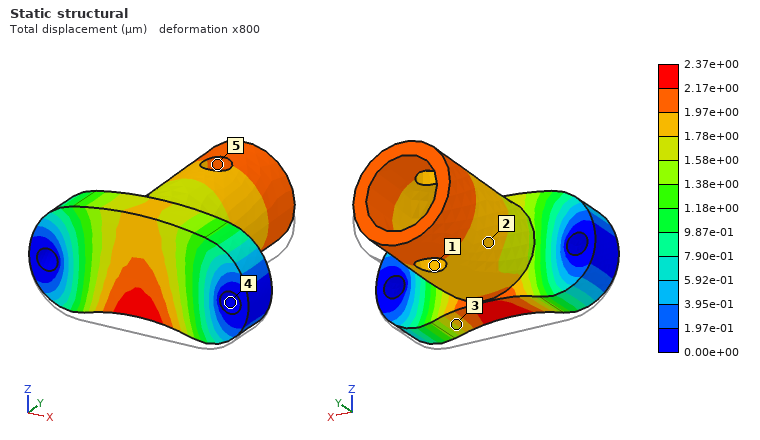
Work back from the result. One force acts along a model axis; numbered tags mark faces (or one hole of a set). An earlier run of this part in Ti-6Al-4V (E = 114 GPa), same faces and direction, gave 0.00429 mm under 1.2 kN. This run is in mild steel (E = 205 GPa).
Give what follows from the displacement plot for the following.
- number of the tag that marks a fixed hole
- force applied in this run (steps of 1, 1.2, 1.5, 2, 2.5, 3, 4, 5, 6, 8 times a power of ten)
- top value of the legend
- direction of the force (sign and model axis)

4
1.2 kN
2.37e+00 µm
+Z
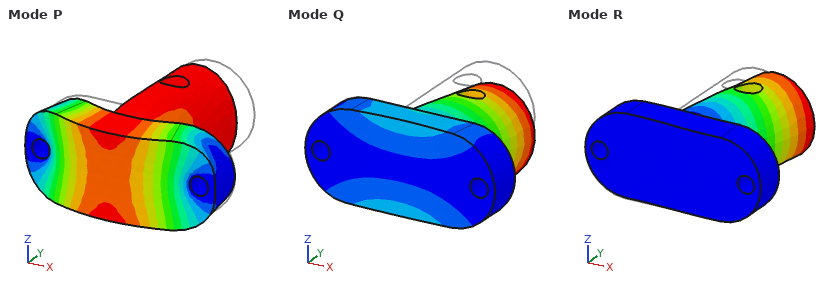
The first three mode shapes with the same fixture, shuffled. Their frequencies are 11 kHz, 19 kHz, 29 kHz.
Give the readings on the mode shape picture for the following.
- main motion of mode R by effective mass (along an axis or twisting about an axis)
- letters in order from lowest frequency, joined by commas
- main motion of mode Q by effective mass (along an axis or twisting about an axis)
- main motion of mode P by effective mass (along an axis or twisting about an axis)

along X
Q, R, P
along Z
along Y
